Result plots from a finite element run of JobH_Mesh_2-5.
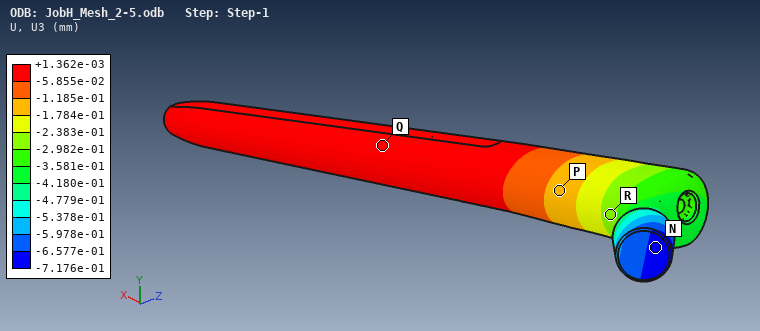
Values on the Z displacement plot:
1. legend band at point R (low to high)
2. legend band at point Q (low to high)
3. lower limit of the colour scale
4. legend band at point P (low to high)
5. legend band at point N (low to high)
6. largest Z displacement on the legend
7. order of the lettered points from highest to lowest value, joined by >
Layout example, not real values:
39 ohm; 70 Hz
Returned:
-2.982e-01 to -2.383e-01 mm; -5.855e-02 to +1.362e-03 mm; -7.176e-01 mm; -1.784e-01 to -1.185e-01 mm; -7.176e-01 to -6.577e-01 mm; +1.362e-03 mm; Q > P > R > N
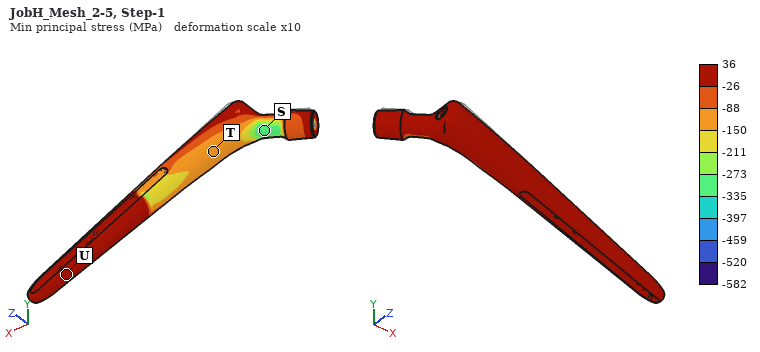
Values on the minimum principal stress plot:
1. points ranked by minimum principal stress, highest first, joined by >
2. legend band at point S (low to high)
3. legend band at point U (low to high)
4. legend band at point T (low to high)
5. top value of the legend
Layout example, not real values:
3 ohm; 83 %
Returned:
U > T > S; -335 to -273 MPa; -26 to 36 MPa; -150 to -88 MPa; 36 MPa
